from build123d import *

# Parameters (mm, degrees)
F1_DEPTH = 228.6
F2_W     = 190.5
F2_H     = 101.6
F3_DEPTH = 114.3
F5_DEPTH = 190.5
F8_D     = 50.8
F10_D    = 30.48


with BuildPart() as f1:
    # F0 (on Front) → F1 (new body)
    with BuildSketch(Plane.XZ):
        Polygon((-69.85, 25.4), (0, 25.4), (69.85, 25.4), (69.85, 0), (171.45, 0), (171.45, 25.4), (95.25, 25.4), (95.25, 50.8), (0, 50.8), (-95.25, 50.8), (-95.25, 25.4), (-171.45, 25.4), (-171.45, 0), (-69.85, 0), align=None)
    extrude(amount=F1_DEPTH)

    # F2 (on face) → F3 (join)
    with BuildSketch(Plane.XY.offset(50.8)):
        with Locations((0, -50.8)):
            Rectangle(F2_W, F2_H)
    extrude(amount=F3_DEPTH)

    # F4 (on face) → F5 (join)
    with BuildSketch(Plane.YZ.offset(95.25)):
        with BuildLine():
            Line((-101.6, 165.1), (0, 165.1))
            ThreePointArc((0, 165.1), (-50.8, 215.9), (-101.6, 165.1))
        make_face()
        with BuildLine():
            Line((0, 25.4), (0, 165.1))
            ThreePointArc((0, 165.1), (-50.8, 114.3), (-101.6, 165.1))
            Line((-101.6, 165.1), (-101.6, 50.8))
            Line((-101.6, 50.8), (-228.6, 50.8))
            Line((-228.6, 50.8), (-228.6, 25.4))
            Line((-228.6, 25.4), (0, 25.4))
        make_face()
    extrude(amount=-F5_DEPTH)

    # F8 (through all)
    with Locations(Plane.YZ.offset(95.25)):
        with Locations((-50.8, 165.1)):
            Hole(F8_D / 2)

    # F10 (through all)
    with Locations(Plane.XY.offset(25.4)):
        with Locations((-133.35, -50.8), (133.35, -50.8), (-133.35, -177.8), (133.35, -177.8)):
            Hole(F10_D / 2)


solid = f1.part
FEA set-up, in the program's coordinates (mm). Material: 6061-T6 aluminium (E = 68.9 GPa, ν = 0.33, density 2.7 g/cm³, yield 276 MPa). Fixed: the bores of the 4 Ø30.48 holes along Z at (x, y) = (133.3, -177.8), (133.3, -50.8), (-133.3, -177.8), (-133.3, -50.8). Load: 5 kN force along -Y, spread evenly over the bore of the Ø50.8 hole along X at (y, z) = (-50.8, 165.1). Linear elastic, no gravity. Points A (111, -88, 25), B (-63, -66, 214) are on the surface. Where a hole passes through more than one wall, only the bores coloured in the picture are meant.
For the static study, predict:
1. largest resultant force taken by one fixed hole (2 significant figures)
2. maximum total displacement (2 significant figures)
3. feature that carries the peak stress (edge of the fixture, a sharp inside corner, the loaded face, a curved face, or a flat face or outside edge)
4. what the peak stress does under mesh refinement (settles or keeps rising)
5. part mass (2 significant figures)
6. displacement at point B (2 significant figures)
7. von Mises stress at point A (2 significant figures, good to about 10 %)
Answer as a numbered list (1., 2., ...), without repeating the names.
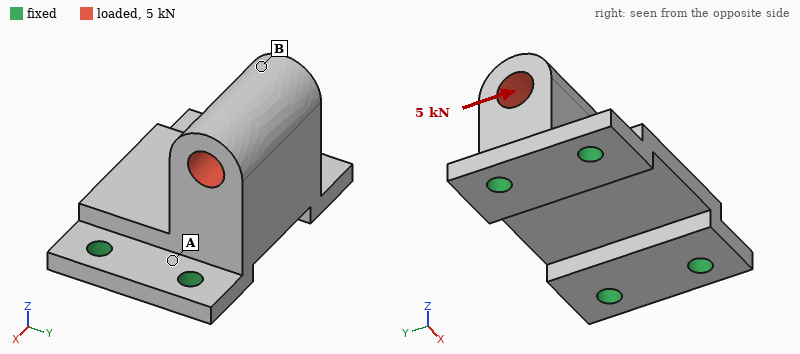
1. 4.6 kN
2. 49 µm
3. edge of the fixture
4. keeps rising
5. 13 kg
6. 49 µm
7. 2.8 MPa
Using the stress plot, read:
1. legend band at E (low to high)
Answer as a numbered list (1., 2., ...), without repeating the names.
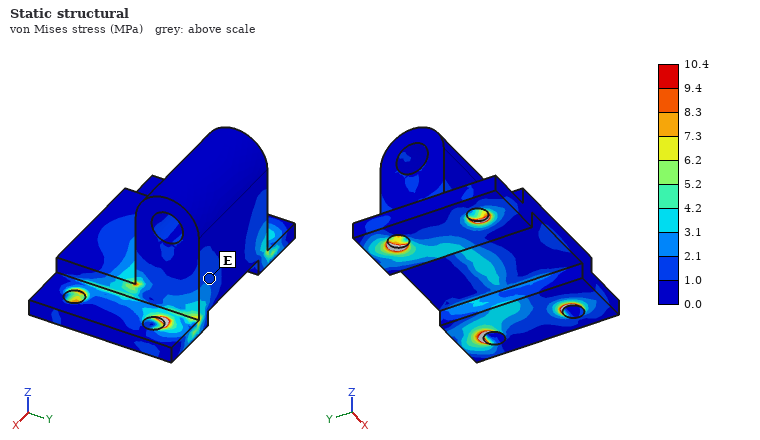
1. 1.0 to 2.1 MPa
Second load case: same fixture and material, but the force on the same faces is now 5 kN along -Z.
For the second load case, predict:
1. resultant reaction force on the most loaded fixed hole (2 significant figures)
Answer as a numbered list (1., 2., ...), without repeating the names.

1. 2.9 kN
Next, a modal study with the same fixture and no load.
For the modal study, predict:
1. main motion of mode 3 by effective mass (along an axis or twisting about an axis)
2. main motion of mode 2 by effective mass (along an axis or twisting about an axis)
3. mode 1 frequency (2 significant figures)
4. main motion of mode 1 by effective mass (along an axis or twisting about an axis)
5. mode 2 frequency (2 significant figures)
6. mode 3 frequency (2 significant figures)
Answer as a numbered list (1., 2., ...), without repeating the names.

1. along Z
2. along X
3. 860 Hz
4. along Y
5. 1600 Hz
6. 1900 Hz
